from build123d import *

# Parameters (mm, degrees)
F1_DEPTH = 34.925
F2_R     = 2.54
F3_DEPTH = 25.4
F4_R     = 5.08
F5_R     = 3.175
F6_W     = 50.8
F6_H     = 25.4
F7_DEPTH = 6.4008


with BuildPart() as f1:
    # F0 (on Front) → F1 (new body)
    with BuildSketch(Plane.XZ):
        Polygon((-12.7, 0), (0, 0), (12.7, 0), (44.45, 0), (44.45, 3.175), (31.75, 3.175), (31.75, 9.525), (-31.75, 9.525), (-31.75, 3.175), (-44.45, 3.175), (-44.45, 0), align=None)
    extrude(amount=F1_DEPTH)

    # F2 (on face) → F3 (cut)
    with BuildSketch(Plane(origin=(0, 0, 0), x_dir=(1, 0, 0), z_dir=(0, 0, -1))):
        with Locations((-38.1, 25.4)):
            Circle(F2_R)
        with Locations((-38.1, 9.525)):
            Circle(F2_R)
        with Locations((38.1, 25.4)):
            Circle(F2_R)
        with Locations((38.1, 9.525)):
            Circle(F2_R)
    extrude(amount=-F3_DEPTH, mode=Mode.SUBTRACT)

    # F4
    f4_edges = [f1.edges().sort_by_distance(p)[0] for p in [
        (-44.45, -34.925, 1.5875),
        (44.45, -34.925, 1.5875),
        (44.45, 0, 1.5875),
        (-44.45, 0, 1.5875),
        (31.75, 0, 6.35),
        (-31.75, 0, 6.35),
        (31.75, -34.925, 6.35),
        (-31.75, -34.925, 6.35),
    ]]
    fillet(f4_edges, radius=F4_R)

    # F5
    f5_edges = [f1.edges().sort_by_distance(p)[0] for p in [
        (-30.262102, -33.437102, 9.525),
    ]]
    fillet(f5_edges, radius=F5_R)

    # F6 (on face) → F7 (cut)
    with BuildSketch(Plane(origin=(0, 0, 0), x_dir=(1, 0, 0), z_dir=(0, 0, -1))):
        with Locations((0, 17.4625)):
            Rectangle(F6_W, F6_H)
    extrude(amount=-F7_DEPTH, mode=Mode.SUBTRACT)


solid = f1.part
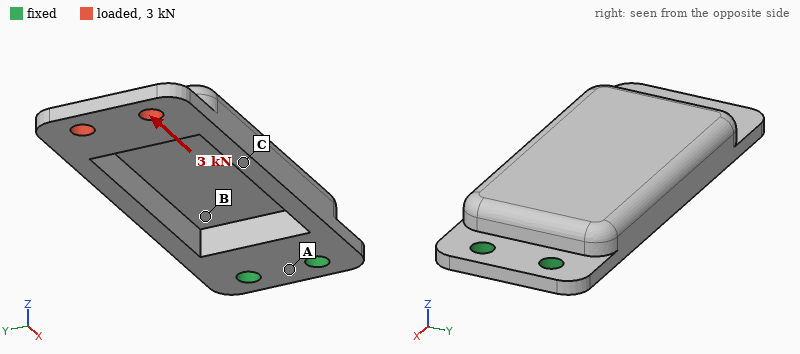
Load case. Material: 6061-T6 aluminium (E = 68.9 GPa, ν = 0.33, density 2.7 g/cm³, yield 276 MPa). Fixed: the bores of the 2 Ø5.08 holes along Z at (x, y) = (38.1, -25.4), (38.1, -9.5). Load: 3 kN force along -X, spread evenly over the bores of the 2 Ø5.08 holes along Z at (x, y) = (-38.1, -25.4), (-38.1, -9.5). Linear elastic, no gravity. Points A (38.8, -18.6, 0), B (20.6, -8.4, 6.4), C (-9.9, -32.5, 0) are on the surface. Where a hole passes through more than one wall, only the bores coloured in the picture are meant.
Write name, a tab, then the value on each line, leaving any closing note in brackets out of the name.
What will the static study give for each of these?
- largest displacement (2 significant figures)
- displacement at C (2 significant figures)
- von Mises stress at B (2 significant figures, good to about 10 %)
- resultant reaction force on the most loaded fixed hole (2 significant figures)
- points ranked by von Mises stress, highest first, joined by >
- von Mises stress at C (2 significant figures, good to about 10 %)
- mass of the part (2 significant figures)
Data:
largest displacement	0.57 mm
displacement at C	0.18 mm
von Mises stress at B	28 MPa
resultant reaction force on the most loaded fixed hole	1.5 kN
points ranked by von Mises stress, highest first, joined by >	C > B > A
von Mises stress at C	94 MPa
mass of the part	40 g
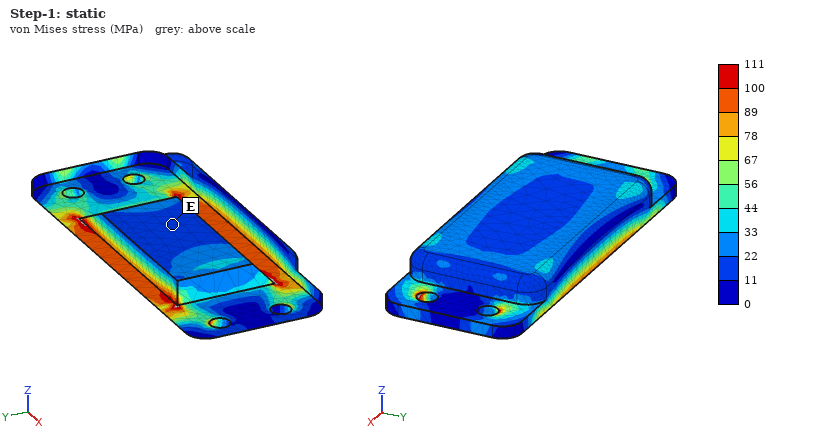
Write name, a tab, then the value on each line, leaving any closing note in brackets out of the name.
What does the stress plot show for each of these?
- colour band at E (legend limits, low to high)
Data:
colour band at E	11 to 22 MPa
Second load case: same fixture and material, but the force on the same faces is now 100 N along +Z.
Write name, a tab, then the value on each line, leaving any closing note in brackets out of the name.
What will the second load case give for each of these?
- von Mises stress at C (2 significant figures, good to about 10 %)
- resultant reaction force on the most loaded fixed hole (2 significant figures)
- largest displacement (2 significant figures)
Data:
von Mises stress at C	15 MPa
resultant reaction force on the most loaded fixed hole	150 N
largest displacement	0.76 mm
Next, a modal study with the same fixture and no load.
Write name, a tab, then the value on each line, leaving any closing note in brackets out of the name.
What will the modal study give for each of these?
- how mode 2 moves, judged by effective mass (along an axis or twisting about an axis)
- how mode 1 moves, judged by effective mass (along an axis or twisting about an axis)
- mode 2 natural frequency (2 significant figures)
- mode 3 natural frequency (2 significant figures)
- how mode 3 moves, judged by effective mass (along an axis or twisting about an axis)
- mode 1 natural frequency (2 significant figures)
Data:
how mode 2 moves, judged by effective mass	along Y
how mode 1 moves, judged by effective mass	along Z
mode 2 natural frequency	1800 Hz
mode 3 natural frequency	3700 Hz
how mode 3 moves, judged by effective mass	along Y
mode 1 natural frequency	540 Hz
